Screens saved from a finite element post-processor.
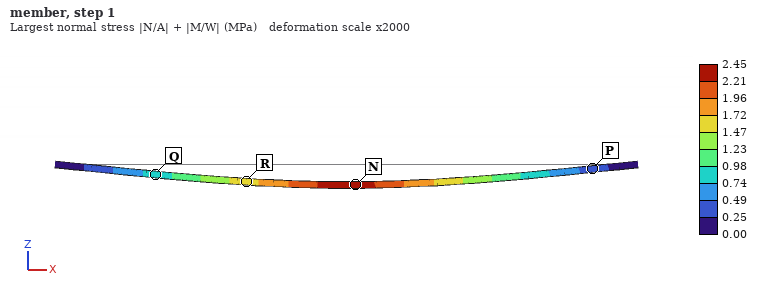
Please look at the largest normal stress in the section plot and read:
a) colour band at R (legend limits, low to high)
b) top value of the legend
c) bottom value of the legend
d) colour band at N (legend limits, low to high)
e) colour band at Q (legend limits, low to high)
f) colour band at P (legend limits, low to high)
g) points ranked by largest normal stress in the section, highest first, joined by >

1.47 to 1.72 MPa
2.45 MPa
0.00 MPa
2.21 to 2.45 MPa
0.74 to 0.98 MPa
0.25 to 0.49 MPa
N > R > Q > P
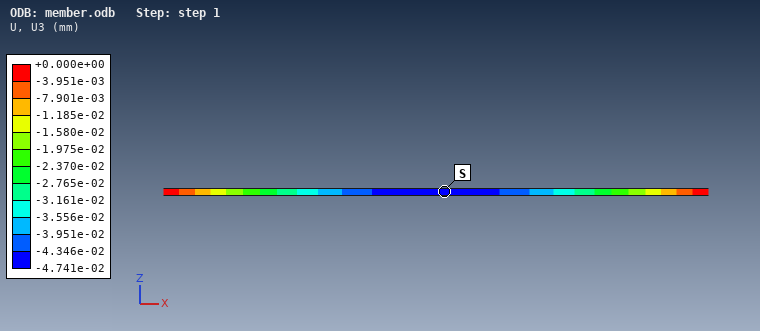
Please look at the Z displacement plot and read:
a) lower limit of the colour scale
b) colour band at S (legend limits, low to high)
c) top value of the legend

-4.741e-02 mm
-4.741e-02 to -4.346e-02 mm
+0.000e+00 mm
